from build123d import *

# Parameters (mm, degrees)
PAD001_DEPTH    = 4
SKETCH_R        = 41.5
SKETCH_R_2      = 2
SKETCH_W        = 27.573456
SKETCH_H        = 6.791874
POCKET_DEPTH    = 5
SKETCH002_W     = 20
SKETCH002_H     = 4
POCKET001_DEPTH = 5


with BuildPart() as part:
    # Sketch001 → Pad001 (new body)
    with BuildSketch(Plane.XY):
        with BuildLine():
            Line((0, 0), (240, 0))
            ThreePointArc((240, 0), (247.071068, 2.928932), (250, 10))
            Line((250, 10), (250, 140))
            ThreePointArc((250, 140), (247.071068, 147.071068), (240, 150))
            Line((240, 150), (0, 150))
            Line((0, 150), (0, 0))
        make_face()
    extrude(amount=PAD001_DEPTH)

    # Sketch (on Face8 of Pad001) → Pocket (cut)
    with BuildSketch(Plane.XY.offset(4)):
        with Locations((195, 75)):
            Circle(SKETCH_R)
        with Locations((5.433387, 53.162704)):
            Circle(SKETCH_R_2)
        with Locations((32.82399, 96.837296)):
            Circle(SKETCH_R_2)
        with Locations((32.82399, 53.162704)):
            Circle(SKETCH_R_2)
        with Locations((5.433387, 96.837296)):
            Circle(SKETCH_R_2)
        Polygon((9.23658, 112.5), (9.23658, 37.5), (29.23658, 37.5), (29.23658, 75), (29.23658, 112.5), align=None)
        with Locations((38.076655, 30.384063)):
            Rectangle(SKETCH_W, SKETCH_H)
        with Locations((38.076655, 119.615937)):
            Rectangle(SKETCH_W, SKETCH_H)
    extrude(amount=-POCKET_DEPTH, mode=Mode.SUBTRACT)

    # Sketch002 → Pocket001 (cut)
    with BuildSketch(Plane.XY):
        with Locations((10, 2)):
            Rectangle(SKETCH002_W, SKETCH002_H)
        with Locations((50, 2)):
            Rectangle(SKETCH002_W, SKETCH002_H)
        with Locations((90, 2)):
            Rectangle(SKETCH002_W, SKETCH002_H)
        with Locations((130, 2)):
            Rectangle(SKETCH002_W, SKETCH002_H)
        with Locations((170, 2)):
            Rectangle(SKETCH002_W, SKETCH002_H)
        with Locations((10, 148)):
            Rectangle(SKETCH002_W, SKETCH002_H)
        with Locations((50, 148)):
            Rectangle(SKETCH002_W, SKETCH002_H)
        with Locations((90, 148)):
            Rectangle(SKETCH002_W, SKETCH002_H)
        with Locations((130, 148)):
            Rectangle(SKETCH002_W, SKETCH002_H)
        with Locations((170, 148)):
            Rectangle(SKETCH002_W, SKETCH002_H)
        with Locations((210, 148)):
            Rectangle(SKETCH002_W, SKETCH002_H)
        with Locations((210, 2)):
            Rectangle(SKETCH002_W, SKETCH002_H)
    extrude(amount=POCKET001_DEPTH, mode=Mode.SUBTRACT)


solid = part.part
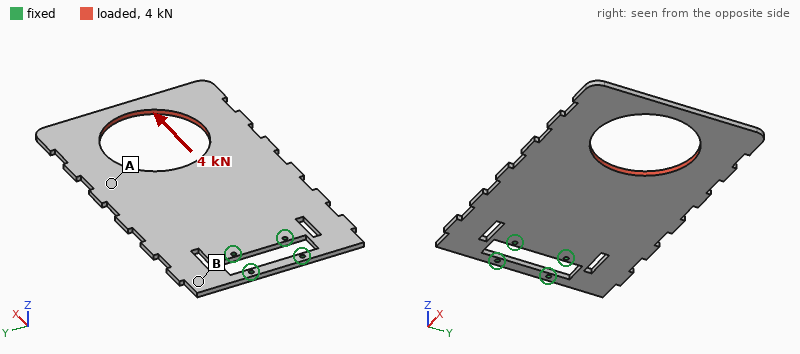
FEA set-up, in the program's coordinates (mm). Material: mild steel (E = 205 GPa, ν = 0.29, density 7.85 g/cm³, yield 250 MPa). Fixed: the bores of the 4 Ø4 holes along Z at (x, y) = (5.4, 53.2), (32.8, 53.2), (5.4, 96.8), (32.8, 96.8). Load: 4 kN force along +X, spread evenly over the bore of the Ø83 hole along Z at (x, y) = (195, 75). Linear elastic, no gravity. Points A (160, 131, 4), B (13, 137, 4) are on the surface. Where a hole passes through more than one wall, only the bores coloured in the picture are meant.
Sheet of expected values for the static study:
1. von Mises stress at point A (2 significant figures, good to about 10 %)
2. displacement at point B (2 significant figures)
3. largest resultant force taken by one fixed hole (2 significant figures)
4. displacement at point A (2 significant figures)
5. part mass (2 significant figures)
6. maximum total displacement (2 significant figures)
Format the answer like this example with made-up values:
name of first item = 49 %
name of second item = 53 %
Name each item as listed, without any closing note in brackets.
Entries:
von Mises stress at point A = 11 MPa
displacement at point B = 4.2 µm
largest resultant force taken by one fixed hole = 1.9 kN
displacement at point A = 8.6 µm
part mass = 920 g
maximum total displacement = 22 µm
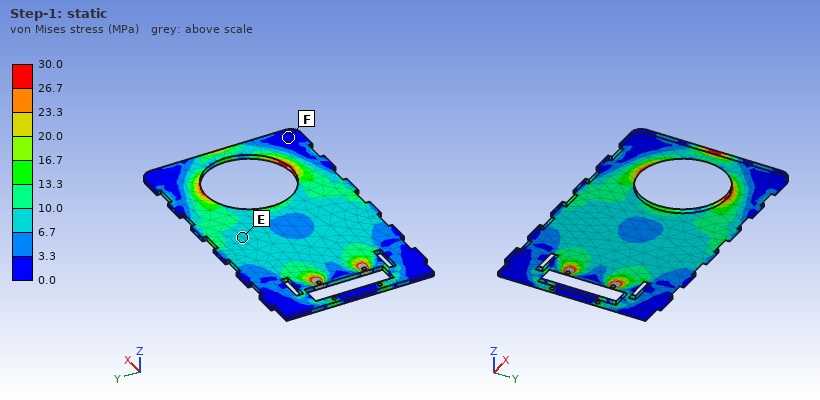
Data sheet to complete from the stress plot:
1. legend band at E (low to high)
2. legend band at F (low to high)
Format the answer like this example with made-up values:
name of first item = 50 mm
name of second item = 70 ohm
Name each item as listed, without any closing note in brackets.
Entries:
legend band at E = 6.7 to 10.0 MPa
legend band at F = 0.0 to 3.3 MPa
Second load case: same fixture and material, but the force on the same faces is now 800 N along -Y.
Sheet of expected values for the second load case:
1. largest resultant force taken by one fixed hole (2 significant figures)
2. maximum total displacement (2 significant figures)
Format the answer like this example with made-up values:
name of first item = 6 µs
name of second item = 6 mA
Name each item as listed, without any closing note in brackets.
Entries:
largest resultant force taken by one fixed hole = 2.2 kN
maximum total displacement = 57 µm
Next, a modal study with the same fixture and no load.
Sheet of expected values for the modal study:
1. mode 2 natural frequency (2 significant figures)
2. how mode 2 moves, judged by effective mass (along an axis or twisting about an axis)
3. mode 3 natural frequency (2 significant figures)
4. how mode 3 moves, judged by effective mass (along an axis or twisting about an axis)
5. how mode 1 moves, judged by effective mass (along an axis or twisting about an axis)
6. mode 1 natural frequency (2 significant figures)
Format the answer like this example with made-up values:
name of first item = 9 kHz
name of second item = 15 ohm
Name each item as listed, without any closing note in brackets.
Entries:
mode 2 natural frequency = 200 Hz
how mode 2 moves, judged by effective mass = twisting about X
mode 3 natural frequency = 360 Hz
how mode 3 moves, judged by effective mass = along Z
how mode 1 moves, judged by effective mass = along Z
mode 1 natural frequency = 75 Hz
